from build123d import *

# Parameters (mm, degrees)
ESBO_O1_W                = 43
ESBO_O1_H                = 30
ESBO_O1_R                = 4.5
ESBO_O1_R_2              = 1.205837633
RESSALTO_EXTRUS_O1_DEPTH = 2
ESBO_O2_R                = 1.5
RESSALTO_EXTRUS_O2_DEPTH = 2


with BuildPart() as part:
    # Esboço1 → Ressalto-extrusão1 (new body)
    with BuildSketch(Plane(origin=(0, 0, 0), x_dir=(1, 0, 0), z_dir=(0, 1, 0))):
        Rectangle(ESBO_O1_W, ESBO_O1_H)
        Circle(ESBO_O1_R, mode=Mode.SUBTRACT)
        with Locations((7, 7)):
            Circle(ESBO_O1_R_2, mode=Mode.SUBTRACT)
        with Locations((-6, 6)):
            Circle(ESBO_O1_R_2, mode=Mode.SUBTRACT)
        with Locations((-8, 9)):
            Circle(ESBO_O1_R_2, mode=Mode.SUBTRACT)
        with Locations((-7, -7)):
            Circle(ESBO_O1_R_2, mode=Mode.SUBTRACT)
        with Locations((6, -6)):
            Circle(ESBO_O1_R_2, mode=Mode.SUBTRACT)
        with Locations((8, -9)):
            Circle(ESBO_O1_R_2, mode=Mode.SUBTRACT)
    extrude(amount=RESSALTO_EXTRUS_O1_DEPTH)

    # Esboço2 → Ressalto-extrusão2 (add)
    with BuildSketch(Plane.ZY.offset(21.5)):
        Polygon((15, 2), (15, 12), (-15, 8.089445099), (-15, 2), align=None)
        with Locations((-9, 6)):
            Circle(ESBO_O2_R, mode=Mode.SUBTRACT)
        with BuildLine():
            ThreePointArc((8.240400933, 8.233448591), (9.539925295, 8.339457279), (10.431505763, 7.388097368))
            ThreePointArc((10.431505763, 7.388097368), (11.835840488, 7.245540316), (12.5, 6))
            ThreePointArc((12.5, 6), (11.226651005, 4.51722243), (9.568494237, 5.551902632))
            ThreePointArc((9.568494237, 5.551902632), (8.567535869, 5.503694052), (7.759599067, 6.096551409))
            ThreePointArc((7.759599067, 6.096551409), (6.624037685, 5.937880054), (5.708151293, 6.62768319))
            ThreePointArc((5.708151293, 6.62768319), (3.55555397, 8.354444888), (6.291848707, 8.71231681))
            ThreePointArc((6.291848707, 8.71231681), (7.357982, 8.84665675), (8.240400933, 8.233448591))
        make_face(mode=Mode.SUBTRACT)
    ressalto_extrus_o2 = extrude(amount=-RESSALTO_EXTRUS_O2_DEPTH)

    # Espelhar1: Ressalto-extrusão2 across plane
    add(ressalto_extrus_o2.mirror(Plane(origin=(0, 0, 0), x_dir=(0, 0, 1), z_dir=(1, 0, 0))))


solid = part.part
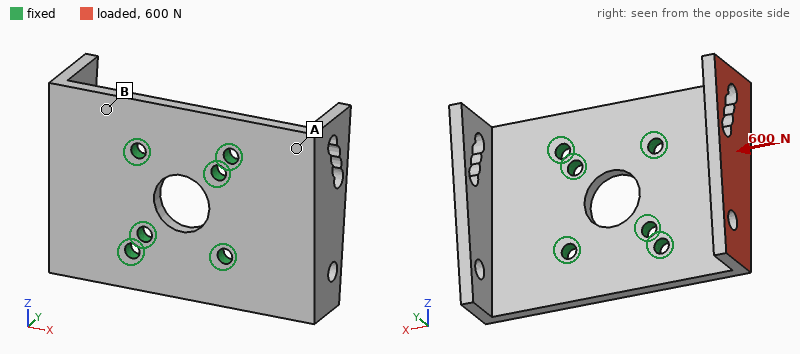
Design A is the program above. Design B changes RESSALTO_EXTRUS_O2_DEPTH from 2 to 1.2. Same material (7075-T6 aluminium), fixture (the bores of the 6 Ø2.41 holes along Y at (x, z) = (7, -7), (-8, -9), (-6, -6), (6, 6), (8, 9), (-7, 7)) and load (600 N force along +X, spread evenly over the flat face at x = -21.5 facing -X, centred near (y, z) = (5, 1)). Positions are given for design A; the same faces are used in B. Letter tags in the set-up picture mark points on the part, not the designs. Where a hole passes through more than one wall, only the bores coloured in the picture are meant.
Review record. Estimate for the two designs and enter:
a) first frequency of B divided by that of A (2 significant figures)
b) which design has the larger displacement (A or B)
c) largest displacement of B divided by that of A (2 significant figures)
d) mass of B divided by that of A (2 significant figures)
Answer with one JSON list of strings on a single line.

["1.1", "B", "1.7", "0.90"]
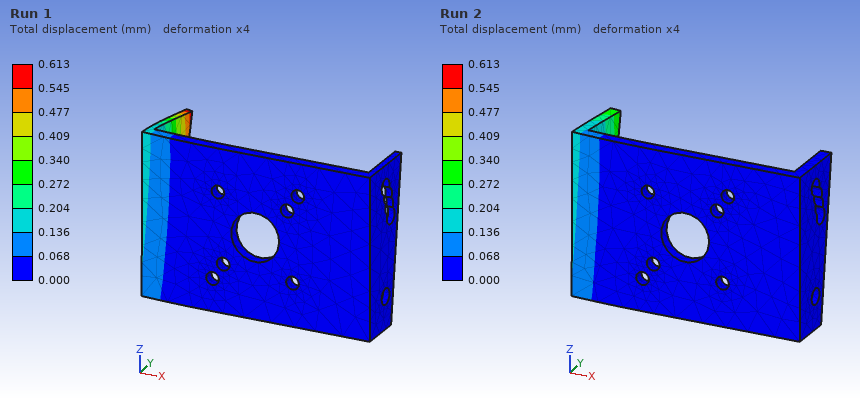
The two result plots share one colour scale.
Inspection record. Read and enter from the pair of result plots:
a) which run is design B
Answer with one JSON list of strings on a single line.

["Run 1"]
